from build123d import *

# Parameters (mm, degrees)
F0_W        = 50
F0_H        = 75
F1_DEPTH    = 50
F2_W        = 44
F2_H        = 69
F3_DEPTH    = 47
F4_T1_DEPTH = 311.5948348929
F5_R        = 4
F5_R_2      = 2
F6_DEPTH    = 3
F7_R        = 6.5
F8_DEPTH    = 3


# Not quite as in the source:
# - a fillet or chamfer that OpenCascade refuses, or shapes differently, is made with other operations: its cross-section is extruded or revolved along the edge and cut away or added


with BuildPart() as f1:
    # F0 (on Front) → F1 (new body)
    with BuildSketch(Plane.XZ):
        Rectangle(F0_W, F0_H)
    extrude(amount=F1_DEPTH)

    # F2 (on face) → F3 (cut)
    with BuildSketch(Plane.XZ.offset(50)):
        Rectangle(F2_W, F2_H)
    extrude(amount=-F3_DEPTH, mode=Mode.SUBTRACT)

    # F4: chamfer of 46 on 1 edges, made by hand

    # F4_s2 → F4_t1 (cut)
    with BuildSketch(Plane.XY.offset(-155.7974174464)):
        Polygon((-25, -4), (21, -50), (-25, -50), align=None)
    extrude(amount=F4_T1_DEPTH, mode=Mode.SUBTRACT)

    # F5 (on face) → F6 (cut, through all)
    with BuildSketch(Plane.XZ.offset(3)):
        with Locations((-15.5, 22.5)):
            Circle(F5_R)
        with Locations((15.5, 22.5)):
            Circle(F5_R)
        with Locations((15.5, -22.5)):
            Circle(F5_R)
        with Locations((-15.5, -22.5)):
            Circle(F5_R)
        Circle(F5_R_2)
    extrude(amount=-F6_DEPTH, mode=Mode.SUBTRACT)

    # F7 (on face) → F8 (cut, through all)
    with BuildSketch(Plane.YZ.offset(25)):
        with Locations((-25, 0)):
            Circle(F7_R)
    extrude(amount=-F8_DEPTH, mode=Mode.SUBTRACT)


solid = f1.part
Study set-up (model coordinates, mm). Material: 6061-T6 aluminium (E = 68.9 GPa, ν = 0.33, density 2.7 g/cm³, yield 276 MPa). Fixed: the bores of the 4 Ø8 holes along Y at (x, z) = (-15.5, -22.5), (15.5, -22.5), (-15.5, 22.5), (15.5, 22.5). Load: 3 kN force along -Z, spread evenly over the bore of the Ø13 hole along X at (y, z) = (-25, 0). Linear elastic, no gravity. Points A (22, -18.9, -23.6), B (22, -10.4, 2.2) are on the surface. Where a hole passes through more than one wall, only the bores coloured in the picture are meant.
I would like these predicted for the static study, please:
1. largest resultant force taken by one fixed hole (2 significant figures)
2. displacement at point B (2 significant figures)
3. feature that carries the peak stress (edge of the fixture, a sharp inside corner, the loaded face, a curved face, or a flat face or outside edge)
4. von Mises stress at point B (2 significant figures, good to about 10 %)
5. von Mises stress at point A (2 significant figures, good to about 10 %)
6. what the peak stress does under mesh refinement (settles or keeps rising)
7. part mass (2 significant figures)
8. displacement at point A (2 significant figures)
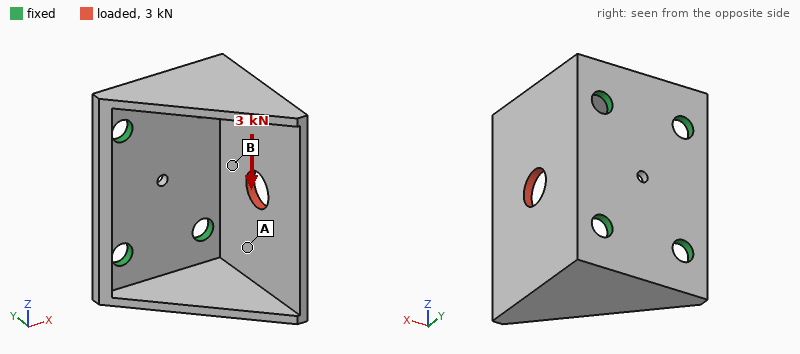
2.1 kN
19 µm
edge of the fixture
49 MPa
23 MPa
keeps rising
76 g
42 µm
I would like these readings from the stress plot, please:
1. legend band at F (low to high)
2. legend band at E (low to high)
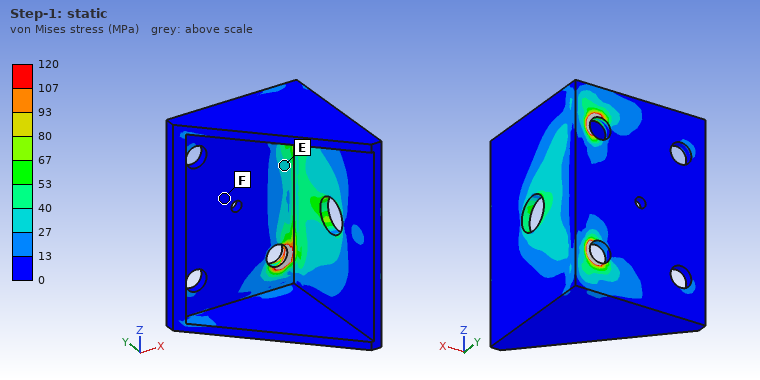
0 to 13 MPa
27 to 40 MPa
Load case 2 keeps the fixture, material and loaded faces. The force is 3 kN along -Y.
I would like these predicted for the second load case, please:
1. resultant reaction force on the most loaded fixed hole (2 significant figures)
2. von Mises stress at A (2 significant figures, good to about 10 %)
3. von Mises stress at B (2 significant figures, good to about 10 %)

1.6 kN
16 MPa
20 MPa
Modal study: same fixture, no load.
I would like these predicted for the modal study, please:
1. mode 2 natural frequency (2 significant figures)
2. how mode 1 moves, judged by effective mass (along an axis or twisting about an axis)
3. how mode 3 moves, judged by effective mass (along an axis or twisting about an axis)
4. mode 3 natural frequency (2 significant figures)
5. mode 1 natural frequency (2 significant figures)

4200 Hz
along X
along Z
4700 Hz
2200 Hz
